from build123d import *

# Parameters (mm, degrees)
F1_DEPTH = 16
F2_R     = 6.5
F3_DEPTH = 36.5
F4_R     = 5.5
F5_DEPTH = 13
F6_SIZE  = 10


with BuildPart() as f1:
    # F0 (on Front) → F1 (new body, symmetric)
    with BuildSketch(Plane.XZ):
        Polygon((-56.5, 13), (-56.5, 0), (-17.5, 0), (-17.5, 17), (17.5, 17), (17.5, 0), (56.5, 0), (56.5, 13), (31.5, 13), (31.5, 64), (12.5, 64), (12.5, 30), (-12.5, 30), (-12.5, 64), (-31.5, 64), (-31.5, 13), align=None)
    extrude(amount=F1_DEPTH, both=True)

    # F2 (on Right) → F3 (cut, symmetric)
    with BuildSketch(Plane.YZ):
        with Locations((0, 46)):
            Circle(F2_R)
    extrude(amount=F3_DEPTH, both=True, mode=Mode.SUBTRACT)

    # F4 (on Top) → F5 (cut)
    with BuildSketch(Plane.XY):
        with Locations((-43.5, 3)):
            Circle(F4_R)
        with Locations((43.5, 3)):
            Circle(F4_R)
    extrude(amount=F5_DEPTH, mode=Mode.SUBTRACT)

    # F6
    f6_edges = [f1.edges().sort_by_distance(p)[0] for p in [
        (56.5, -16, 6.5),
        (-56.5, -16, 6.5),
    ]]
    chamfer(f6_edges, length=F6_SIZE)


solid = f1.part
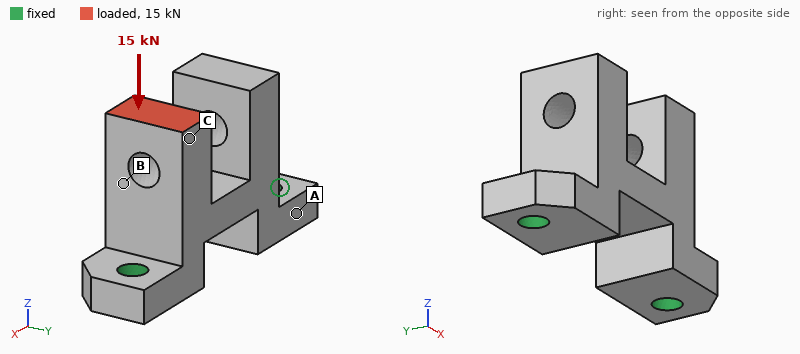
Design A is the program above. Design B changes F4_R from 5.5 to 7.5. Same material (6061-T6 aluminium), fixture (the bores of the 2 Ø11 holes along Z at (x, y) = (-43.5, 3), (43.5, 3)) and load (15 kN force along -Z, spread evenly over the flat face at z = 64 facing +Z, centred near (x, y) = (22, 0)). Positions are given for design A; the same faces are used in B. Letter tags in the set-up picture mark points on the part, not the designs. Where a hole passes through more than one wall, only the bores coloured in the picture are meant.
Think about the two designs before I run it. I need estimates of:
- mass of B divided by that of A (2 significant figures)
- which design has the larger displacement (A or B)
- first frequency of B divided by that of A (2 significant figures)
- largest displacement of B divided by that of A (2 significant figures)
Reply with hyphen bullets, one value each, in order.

- 0.98
- A
- 1.1
- 0.82
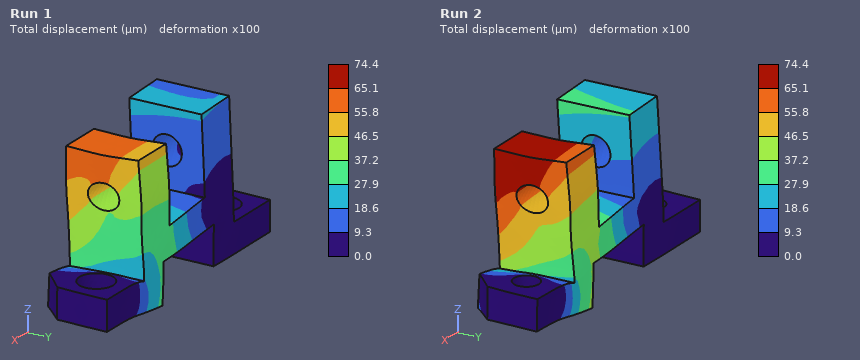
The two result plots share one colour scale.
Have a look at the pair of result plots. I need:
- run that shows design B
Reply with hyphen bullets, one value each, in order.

- Run 1
